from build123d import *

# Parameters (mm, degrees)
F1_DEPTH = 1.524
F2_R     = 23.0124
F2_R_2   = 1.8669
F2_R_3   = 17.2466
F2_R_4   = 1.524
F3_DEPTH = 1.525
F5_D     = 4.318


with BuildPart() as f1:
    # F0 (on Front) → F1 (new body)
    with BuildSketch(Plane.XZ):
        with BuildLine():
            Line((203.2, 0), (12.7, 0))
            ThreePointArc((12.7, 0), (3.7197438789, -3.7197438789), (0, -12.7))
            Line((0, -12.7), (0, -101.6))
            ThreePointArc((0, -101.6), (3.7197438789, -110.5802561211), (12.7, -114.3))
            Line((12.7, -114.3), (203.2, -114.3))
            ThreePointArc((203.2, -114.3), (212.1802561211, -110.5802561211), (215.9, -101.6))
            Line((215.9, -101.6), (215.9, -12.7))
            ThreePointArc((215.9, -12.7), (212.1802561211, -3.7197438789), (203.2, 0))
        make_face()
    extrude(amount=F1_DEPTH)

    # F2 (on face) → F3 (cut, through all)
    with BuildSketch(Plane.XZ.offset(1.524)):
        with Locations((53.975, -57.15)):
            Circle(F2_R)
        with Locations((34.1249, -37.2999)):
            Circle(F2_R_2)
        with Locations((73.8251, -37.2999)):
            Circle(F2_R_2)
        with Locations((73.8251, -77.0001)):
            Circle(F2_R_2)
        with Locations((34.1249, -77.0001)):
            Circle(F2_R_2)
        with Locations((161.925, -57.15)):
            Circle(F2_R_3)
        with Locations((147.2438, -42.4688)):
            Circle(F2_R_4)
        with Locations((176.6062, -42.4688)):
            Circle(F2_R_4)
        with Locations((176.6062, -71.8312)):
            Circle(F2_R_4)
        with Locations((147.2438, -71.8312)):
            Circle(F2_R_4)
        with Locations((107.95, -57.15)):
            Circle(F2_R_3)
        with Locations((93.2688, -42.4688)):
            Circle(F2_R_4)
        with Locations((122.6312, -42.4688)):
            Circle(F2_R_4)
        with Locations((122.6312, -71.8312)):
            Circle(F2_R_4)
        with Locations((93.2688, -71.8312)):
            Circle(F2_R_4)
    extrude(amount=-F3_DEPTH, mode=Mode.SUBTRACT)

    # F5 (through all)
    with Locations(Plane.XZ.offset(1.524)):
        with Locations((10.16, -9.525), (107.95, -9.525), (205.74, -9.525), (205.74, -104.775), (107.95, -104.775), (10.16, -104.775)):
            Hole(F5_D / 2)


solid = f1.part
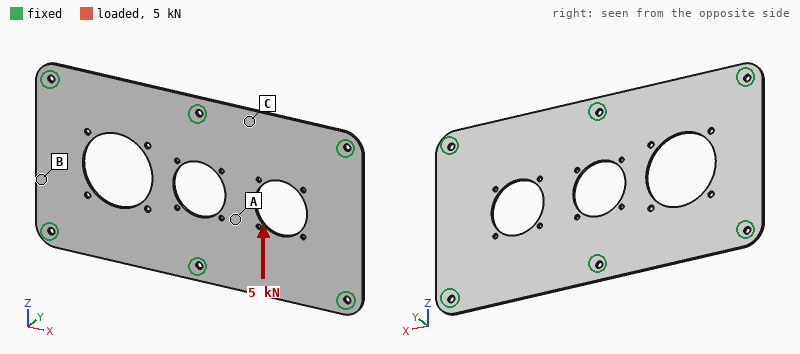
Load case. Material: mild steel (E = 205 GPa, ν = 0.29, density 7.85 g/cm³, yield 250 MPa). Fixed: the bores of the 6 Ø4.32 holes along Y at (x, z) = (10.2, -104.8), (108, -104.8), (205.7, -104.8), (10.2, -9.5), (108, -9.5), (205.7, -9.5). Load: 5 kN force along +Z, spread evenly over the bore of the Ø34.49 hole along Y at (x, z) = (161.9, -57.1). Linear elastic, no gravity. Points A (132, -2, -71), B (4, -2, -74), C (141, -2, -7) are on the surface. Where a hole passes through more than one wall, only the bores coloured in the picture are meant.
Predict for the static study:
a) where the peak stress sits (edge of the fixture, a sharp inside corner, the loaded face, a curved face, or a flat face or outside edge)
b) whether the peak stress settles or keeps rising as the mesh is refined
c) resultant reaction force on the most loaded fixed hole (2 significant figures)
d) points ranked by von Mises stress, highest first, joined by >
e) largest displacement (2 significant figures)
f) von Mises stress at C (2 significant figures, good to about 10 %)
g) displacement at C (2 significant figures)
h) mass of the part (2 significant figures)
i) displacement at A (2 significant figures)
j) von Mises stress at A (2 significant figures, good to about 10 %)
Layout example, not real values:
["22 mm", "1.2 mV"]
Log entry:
["edge of the fixture", "keeps rising", "1.6 kN", "A > C > B", "14 µm", "14 MPa", "10 µm", "250 g", "9.5 µm", "26 MPa"]
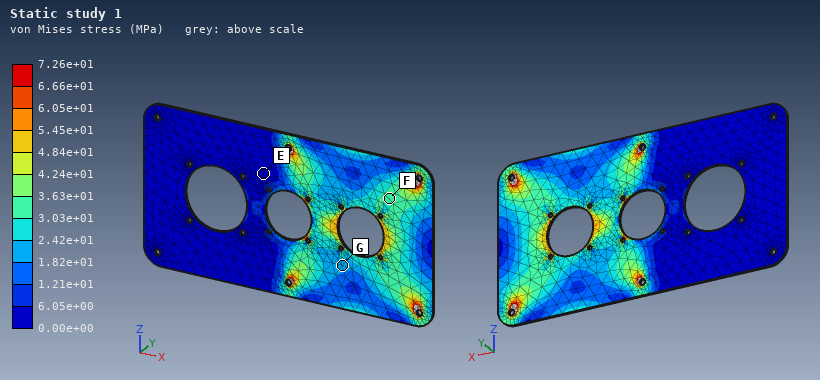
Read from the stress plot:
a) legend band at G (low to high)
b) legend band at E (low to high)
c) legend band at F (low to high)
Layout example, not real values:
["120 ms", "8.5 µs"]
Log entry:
["1.82e+01 to 2.42e+01 MPa", "0.00e+00 to 6.05e+00 MPa", "3.03e+01 to 3.63e+01 MPa"]
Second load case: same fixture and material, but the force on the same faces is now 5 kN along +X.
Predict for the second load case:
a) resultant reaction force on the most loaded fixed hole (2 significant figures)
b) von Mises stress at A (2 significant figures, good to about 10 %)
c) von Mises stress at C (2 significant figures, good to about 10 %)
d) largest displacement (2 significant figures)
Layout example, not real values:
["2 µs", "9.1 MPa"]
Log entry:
["1.3 kN", "33 MPa", "11 MPa", "13 µm"]
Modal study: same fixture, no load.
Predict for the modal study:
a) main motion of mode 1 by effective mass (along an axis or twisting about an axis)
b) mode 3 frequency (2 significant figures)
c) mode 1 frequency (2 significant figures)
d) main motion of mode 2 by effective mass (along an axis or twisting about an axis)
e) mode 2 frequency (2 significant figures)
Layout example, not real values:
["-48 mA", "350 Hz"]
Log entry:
["along Y", "900 Hz", "600 Hz", "along Y", "640 Hz"]
